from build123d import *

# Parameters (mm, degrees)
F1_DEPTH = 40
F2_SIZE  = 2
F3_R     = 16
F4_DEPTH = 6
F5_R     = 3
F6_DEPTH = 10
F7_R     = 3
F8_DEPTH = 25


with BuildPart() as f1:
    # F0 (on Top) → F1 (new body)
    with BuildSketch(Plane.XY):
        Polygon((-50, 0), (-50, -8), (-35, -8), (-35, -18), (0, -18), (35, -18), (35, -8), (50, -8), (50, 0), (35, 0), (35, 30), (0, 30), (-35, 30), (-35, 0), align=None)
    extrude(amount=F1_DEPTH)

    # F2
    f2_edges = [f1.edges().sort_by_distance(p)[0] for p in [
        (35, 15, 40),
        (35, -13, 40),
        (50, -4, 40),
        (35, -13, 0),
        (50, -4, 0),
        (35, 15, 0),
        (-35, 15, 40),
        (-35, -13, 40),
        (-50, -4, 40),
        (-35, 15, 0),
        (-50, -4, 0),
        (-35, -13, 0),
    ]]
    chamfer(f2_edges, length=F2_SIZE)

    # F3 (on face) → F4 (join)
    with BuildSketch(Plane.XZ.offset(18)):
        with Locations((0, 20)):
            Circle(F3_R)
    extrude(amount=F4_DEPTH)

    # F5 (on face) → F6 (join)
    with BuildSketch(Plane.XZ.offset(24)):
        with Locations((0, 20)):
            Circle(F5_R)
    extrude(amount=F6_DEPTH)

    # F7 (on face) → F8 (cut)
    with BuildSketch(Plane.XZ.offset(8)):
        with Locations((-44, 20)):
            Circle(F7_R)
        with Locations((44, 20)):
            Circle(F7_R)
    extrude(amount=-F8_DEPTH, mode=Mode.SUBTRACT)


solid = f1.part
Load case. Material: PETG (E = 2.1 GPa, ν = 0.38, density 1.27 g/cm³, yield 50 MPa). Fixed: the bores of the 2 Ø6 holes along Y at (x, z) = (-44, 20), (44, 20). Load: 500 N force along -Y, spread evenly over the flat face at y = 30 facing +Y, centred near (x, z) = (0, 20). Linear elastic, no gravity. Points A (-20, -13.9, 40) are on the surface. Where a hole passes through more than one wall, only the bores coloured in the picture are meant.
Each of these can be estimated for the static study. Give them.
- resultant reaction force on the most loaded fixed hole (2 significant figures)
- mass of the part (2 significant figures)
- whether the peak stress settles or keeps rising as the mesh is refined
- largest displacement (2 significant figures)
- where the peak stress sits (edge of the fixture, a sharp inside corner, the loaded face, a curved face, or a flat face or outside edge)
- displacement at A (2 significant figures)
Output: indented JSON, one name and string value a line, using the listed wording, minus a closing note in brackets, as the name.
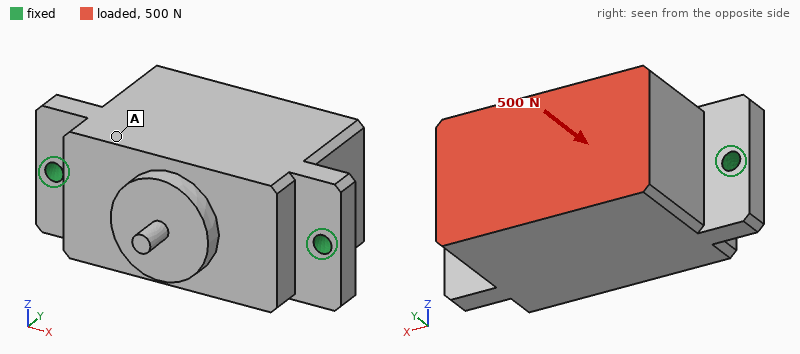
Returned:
{
  "resultant reaction force on the most loaded fixed hole": "250 N",
  "mass of the part": "190 g",
  "whether the peak stress settles or keeps rising as the mesh is refined": "keeps rising",
  "largest displacement": "42 µm",
  "where the peak stress sits": "edge of the fixture",
  "displacement at A": "39 µm"
}
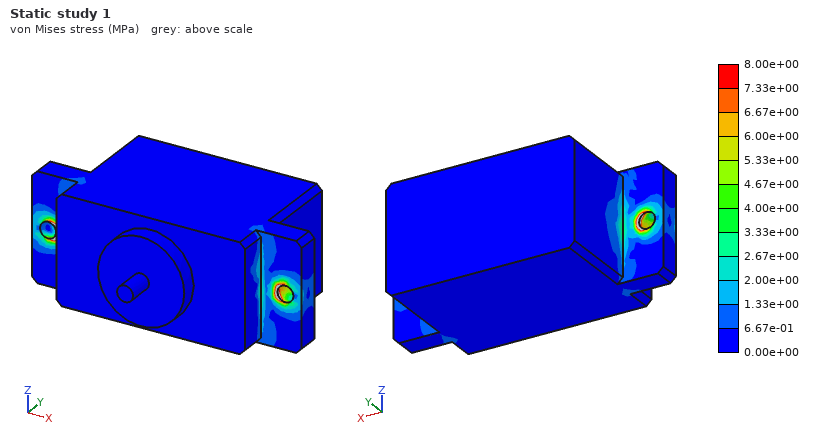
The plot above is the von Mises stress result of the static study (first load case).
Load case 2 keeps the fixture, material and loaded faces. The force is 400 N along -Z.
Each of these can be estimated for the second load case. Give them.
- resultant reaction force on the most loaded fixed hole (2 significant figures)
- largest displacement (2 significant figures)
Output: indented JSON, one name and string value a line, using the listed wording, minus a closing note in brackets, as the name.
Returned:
{
  "resultant reaction force on the most loaded fixed hole": "200 N",
  "largest displacement": "0.69 mm"
}
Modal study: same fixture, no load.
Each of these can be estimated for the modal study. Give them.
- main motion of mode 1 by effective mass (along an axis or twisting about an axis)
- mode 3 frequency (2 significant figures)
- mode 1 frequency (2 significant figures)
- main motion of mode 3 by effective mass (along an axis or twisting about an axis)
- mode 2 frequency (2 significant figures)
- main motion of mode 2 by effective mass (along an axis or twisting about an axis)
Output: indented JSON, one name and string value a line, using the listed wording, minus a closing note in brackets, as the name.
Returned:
{
  "main motion of mode 1 by effective mass": "along Z",
  "mode 3 frequency": "1700 Hz",
  "mode 1 frequency": "520 Hz",
  "main motion of mode 3 by effective mass": "along Z",
  "mode 2 frequency": "1300 Hz",
  "main motion of mode 2 by effective mass": "along Y"
}
